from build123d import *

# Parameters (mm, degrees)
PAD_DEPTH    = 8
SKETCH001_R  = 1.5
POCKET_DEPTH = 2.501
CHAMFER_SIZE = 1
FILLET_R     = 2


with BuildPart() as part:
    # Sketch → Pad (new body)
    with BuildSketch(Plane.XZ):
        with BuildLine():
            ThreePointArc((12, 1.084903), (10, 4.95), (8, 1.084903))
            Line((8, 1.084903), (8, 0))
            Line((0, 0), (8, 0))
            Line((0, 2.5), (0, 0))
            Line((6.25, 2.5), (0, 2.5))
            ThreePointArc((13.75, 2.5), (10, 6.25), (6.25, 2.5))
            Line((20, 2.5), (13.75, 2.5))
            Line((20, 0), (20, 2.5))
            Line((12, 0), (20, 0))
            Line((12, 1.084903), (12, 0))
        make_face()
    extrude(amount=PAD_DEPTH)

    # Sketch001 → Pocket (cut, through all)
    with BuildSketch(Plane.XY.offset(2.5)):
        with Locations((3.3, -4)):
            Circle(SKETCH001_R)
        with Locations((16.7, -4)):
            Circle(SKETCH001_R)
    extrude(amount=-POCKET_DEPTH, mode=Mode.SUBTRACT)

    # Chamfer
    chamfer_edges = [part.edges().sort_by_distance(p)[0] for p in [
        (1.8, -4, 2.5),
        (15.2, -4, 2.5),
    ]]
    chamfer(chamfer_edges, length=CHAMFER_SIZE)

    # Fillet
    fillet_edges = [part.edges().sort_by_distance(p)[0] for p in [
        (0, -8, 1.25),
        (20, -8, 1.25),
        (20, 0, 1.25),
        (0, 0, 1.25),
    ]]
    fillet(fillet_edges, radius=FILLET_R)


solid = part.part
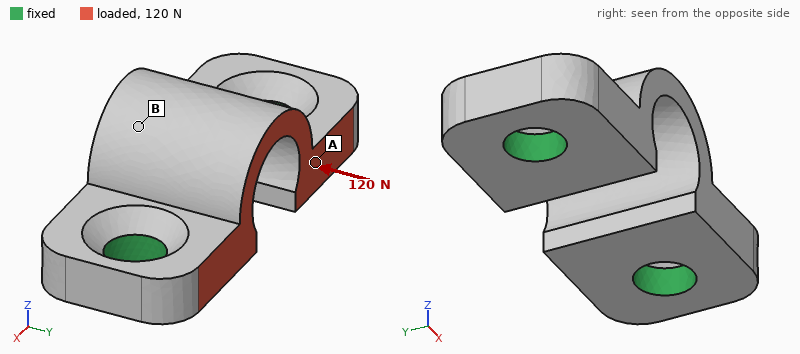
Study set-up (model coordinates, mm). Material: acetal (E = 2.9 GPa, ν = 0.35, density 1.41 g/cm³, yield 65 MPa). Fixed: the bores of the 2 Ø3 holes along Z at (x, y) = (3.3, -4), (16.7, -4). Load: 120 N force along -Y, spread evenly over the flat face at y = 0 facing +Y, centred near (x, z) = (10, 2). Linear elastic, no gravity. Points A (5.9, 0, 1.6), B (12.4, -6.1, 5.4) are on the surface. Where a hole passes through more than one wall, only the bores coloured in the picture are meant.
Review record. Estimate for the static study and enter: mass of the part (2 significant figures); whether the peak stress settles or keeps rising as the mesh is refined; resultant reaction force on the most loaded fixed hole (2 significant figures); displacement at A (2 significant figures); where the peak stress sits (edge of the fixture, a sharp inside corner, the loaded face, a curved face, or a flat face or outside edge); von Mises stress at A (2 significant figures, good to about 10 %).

0.51 g
keeps rising
60 N
31 µm
edge of the fixture
5.4 MPa
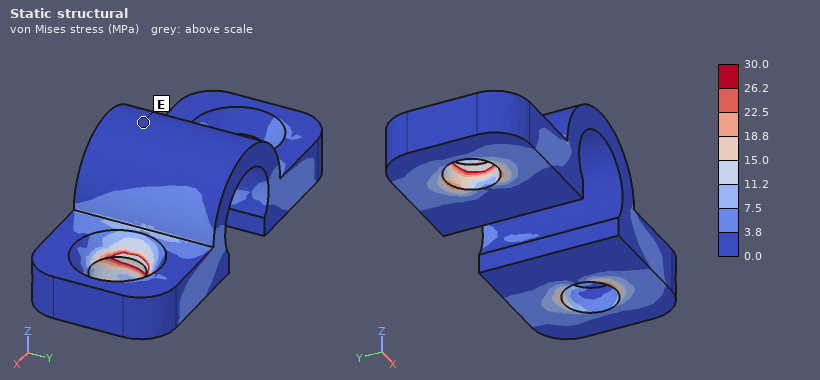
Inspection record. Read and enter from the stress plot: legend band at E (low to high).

0.0 to 3.8 MPa
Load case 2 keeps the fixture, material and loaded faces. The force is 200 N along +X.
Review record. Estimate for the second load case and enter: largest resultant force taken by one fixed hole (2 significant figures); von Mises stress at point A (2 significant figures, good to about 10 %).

100 N
14 MPa
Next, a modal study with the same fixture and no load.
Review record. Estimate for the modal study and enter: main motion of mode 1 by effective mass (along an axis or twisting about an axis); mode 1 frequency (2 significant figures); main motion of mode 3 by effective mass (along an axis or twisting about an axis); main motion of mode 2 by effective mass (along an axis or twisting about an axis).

along Y
11 kHz
along Z
along X
